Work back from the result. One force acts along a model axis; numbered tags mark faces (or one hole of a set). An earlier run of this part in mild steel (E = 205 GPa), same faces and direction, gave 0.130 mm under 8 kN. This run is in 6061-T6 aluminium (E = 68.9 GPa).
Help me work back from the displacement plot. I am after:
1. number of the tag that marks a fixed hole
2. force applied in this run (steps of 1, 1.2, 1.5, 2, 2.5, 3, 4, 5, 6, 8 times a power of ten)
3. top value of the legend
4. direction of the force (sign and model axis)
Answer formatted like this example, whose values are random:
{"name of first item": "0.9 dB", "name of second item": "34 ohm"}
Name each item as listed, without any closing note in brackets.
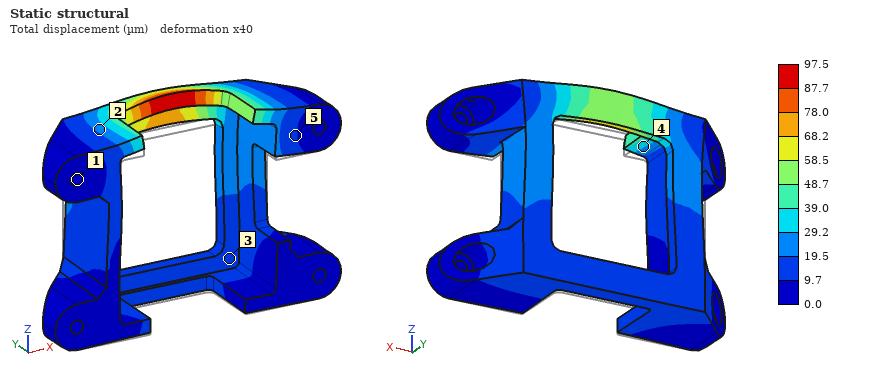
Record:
{"number of the tag that marks a fixed hole": "1", "force applied in this run": "2 kN", "top value of the legend": "97.5 µm", "direction of the force": "+Z"}
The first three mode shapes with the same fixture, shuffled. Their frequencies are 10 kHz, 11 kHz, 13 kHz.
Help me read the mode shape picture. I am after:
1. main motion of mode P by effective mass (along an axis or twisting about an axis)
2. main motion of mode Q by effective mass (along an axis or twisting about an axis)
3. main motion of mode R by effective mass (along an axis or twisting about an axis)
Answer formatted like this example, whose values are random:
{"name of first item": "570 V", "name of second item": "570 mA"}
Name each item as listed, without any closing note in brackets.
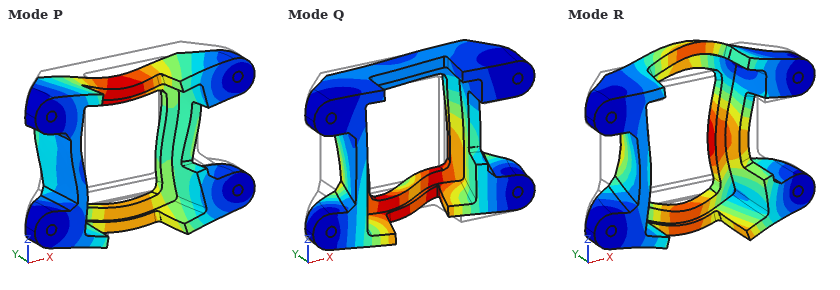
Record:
{"main motion of mode P by effective mass": "along Z", "main motion of mode Q by effective mass": "along X", "main motion of mode R by effective mass": "along Y"}
